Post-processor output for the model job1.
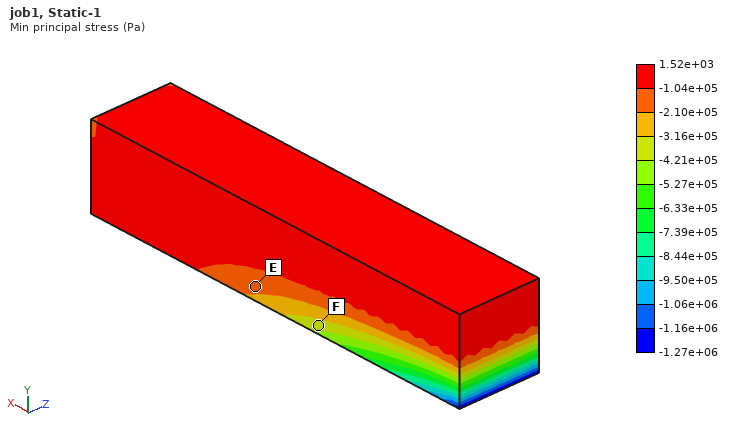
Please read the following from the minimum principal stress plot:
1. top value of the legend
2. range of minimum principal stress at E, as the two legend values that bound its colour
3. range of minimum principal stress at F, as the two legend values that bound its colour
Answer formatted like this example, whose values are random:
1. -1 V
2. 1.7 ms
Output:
1. 1.52e+03 Pa
2. -2.10e+05 to -1.04e+05 Pa
3. -4.21e+05 to -3.16e+05 Pa
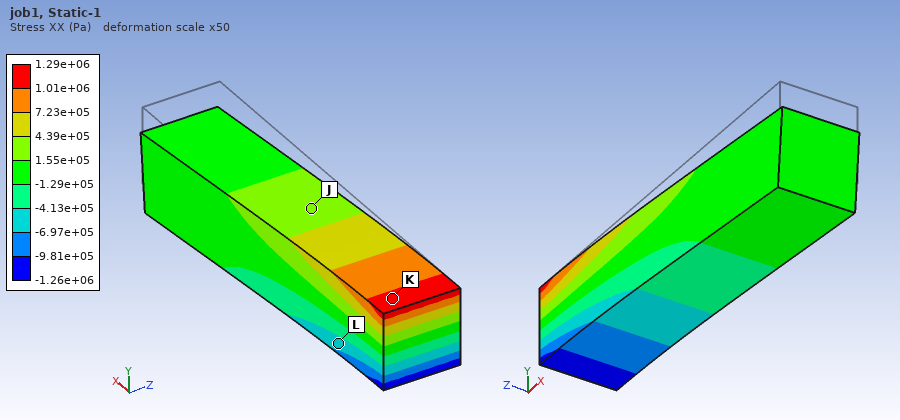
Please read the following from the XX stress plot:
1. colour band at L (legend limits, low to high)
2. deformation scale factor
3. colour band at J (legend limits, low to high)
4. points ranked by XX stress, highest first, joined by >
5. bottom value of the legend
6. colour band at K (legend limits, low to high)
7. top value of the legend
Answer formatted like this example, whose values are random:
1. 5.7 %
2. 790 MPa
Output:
1. -6.97e+05 to -4.13e+05 Pa
2. 50
3. 1.55e+05 to 4.39e+05 Pa
4. K > J > L
5. -1.26e+06 Pa
6. 1.01e+06 to 1.29e+06 Pa
7. 1.29e+06 Pa
